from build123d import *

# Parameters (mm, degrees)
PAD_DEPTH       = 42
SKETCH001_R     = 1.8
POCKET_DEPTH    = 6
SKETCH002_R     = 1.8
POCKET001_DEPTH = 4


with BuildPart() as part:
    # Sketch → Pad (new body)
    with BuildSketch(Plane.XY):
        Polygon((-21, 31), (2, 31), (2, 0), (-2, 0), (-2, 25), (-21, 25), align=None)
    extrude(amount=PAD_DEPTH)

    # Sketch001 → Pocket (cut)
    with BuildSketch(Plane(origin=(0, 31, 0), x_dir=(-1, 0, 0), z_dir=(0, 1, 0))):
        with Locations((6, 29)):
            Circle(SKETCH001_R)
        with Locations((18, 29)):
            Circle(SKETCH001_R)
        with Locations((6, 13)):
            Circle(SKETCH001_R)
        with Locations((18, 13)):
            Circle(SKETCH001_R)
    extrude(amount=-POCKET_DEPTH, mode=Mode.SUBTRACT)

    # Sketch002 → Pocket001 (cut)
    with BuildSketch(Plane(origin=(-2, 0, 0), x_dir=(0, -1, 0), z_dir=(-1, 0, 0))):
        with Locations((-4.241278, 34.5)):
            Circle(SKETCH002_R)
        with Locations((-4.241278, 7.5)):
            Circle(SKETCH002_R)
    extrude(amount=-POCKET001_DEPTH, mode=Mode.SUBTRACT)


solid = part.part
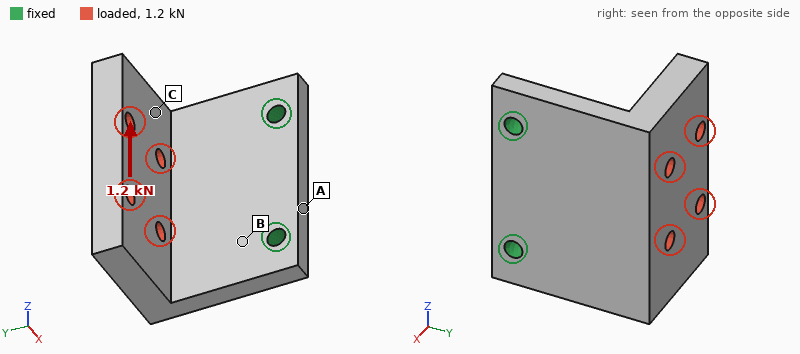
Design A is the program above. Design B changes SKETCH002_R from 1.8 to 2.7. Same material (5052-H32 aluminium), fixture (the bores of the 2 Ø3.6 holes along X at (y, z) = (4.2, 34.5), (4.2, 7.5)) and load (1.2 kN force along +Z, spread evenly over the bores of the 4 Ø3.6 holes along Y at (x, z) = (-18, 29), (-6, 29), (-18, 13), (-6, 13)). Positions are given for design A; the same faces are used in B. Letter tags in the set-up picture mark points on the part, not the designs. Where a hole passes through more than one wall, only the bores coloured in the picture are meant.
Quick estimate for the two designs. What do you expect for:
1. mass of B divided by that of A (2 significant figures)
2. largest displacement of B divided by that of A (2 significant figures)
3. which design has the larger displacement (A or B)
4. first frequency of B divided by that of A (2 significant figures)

0.99
0.89
A
1.1
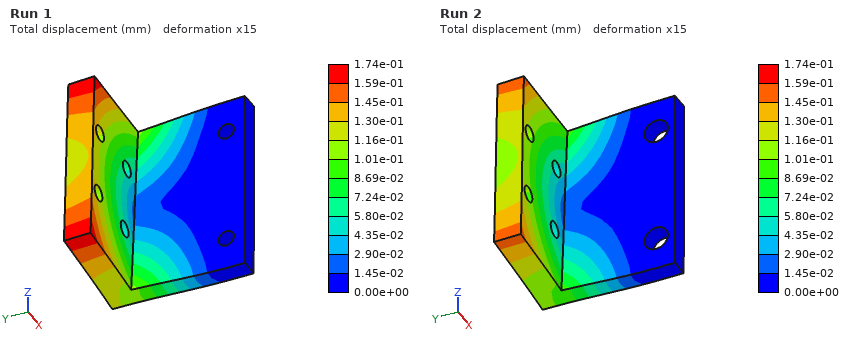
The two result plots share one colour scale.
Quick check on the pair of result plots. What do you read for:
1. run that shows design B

Run 2
